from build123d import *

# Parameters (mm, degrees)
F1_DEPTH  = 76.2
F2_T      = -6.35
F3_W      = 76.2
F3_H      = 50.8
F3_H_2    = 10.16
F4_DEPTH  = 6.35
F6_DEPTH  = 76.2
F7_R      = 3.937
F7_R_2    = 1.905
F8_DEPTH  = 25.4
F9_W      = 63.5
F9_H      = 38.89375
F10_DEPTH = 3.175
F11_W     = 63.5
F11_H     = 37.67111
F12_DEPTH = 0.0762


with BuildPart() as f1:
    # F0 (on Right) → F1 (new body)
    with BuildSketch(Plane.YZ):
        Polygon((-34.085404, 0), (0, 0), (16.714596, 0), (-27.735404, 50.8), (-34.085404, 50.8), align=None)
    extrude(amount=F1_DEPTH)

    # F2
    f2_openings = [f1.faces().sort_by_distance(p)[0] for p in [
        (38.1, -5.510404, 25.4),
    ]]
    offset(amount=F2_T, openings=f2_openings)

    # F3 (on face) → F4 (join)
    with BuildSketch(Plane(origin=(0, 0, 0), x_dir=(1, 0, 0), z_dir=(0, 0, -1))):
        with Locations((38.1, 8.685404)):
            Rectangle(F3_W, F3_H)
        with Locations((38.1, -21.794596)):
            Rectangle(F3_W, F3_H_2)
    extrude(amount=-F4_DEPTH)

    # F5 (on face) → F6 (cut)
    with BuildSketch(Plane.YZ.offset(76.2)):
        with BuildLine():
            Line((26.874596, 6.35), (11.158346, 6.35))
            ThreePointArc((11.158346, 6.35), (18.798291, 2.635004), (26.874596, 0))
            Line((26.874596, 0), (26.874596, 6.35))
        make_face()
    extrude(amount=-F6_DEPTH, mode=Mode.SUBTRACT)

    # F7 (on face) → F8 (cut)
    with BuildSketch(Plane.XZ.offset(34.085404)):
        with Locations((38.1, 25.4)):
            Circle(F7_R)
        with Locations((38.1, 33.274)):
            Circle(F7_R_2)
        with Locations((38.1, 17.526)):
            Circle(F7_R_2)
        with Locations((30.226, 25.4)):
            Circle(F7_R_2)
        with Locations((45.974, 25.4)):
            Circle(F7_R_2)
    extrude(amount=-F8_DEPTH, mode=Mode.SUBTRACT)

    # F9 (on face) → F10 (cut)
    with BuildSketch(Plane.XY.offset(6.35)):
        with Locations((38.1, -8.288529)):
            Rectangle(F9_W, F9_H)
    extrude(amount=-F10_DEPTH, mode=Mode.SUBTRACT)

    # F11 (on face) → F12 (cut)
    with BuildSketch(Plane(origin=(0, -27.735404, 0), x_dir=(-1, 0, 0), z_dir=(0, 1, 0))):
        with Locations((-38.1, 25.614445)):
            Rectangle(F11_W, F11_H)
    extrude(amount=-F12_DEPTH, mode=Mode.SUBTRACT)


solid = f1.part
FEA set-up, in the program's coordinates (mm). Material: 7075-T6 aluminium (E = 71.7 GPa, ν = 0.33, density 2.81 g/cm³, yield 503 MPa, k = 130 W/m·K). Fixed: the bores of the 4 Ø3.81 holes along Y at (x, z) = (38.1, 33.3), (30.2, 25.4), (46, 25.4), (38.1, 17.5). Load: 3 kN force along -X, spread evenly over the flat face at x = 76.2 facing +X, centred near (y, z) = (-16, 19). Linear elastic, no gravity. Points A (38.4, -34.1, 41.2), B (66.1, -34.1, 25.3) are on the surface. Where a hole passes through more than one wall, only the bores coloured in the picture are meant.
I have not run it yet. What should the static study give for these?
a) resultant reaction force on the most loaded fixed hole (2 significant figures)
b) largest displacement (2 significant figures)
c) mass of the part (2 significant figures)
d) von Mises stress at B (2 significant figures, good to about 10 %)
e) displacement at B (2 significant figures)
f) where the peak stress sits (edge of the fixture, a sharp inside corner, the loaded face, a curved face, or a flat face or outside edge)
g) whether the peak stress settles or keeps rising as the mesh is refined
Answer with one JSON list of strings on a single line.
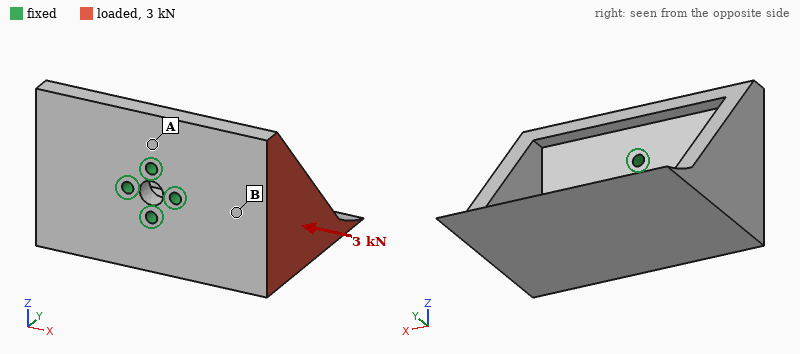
["1.6 kN", "0.27 mm", "140 g", "23 MPa", "0.056 mm", "edge of the fixture", "keeps rising"]
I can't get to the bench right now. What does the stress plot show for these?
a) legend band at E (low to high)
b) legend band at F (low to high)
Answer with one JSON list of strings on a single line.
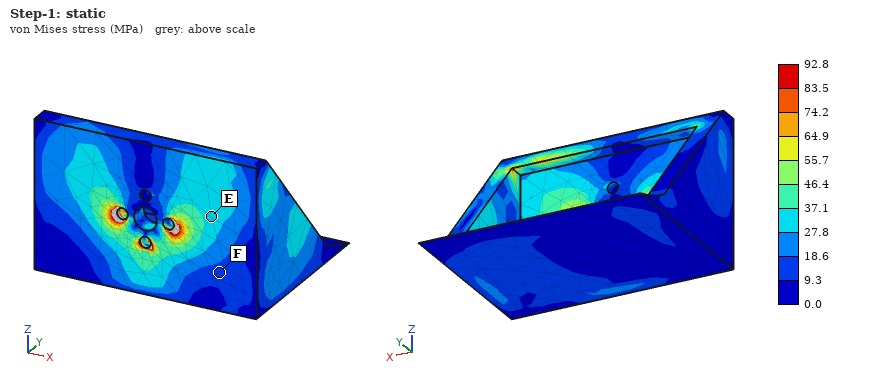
["27.8 to 37.1 MPa", "9.3 to 18.6 MPa"]
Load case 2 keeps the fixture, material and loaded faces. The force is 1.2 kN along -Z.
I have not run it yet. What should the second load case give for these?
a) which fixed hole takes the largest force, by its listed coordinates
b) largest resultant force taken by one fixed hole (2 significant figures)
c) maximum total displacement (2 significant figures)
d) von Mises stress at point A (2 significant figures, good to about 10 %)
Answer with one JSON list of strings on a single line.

["(46, 25.4)", "1.7 kN", "0.16 mm", "26 MPa"]
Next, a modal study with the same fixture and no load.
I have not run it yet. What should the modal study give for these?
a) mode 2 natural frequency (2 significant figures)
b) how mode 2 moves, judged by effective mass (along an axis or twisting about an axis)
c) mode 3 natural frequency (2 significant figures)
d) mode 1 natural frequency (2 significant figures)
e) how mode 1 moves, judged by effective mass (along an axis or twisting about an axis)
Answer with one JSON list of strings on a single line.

["2100 Hz", "along Z", "3100 Hz", "1700 Hz", "along X"]
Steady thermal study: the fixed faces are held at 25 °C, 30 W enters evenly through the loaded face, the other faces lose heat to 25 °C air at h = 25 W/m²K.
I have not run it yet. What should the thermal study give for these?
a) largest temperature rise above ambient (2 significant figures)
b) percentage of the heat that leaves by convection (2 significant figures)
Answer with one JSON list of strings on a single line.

["23 K", "14 %"]
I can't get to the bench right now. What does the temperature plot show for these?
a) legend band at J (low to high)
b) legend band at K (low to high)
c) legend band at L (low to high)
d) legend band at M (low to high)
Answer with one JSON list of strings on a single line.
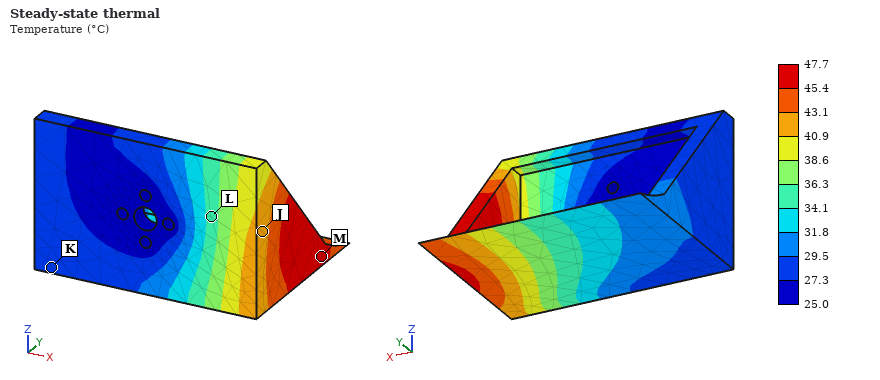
["40.9 to 43.1 °C", "27.3 to 29.5 °C", "34.1 to 36.3 °C", "45.4 to 47.7 °C"]
